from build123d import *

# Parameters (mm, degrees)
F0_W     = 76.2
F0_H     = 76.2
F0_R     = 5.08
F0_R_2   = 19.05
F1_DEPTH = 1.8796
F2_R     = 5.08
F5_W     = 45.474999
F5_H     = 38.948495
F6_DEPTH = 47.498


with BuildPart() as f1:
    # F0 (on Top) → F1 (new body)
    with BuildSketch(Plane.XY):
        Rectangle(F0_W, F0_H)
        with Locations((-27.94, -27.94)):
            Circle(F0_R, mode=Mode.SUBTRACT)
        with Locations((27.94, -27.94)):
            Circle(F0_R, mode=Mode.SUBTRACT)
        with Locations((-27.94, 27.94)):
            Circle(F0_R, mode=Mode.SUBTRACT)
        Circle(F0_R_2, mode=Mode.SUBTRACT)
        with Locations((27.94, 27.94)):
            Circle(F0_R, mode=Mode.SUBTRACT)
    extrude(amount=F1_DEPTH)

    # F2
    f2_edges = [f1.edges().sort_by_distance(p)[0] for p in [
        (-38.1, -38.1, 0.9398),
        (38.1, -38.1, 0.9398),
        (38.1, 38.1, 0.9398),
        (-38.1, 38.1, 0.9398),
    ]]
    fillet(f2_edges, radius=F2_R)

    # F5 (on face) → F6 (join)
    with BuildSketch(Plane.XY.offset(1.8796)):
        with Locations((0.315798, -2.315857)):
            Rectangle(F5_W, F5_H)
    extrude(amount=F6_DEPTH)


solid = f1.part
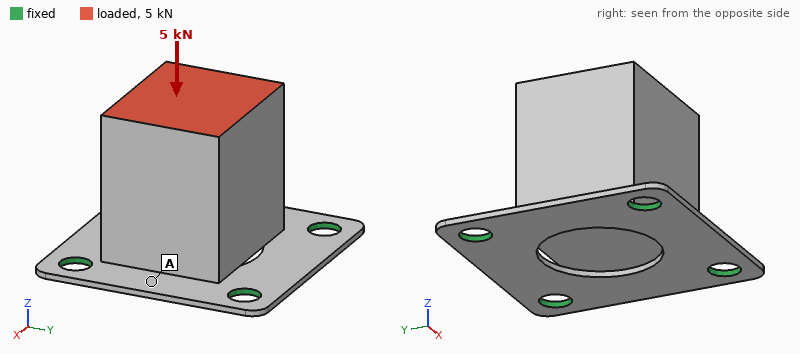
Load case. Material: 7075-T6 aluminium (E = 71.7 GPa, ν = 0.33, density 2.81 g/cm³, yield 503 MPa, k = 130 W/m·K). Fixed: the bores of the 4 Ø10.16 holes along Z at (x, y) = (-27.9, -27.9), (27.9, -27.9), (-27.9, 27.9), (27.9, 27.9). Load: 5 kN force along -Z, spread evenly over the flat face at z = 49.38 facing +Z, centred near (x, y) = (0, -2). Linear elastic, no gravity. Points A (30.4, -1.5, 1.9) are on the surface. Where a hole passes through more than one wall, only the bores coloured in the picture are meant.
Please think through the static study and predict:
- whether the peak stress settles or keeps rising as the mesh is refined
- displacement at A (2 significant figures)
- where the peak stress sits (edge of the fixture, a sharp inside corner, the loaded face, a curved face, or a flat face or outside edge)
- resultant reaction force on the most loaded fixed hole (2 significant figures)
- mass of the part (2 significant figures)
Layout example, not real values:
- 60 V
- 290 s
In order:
- keeps rising
- 0.087 mm
- edge of the fixture
- 1.6 kN
- 260 g
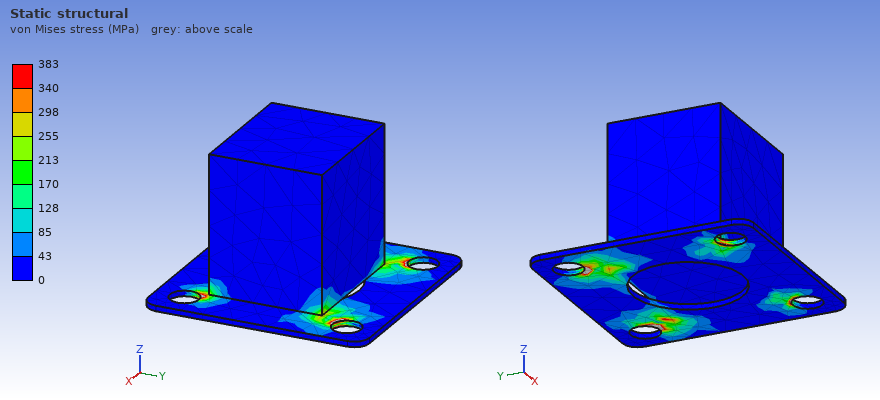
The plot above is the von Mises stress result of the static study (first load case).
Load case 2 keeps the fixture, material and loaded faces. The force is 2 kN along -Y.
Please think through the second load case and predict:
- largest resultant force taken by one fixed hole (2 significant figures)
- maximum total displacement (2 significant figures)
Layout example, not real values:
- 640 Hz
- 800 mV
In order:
- 1.3 kN
- 0.24 mm
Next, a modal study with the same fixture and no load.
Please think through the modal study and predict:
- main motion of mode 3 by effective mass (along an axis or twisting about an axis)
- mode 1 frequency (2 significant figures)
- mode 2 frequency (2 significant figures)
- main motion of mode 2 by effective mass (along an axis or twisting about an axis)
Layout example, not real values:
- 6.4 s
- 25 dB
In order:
- along Z
- 1500 Hz
- 1900 Hz
- along X
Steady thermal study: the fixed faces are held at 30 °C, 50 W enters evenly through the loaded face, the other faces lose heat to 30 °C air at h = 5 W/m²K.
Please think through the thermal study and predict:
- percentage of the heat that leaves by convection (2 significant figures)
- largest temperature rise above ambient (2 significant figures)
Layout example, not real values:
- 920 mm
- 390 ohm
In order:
- 3.6 %
- 34 K
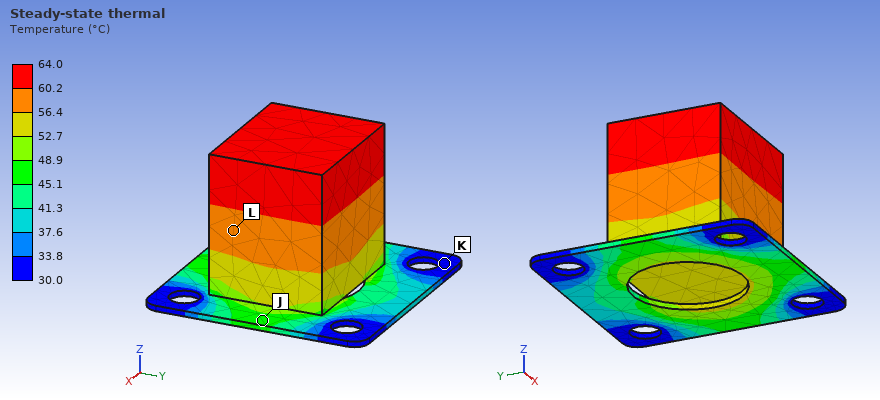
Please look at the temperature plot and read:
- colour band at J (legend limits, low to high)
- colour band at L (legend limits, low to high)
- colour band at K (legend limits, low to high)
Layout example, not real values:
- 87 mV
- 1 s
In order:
- 45.1 to 48.9 °C
- 56.4 to 60.2 °C
- 30.0 to 33.8 °C
